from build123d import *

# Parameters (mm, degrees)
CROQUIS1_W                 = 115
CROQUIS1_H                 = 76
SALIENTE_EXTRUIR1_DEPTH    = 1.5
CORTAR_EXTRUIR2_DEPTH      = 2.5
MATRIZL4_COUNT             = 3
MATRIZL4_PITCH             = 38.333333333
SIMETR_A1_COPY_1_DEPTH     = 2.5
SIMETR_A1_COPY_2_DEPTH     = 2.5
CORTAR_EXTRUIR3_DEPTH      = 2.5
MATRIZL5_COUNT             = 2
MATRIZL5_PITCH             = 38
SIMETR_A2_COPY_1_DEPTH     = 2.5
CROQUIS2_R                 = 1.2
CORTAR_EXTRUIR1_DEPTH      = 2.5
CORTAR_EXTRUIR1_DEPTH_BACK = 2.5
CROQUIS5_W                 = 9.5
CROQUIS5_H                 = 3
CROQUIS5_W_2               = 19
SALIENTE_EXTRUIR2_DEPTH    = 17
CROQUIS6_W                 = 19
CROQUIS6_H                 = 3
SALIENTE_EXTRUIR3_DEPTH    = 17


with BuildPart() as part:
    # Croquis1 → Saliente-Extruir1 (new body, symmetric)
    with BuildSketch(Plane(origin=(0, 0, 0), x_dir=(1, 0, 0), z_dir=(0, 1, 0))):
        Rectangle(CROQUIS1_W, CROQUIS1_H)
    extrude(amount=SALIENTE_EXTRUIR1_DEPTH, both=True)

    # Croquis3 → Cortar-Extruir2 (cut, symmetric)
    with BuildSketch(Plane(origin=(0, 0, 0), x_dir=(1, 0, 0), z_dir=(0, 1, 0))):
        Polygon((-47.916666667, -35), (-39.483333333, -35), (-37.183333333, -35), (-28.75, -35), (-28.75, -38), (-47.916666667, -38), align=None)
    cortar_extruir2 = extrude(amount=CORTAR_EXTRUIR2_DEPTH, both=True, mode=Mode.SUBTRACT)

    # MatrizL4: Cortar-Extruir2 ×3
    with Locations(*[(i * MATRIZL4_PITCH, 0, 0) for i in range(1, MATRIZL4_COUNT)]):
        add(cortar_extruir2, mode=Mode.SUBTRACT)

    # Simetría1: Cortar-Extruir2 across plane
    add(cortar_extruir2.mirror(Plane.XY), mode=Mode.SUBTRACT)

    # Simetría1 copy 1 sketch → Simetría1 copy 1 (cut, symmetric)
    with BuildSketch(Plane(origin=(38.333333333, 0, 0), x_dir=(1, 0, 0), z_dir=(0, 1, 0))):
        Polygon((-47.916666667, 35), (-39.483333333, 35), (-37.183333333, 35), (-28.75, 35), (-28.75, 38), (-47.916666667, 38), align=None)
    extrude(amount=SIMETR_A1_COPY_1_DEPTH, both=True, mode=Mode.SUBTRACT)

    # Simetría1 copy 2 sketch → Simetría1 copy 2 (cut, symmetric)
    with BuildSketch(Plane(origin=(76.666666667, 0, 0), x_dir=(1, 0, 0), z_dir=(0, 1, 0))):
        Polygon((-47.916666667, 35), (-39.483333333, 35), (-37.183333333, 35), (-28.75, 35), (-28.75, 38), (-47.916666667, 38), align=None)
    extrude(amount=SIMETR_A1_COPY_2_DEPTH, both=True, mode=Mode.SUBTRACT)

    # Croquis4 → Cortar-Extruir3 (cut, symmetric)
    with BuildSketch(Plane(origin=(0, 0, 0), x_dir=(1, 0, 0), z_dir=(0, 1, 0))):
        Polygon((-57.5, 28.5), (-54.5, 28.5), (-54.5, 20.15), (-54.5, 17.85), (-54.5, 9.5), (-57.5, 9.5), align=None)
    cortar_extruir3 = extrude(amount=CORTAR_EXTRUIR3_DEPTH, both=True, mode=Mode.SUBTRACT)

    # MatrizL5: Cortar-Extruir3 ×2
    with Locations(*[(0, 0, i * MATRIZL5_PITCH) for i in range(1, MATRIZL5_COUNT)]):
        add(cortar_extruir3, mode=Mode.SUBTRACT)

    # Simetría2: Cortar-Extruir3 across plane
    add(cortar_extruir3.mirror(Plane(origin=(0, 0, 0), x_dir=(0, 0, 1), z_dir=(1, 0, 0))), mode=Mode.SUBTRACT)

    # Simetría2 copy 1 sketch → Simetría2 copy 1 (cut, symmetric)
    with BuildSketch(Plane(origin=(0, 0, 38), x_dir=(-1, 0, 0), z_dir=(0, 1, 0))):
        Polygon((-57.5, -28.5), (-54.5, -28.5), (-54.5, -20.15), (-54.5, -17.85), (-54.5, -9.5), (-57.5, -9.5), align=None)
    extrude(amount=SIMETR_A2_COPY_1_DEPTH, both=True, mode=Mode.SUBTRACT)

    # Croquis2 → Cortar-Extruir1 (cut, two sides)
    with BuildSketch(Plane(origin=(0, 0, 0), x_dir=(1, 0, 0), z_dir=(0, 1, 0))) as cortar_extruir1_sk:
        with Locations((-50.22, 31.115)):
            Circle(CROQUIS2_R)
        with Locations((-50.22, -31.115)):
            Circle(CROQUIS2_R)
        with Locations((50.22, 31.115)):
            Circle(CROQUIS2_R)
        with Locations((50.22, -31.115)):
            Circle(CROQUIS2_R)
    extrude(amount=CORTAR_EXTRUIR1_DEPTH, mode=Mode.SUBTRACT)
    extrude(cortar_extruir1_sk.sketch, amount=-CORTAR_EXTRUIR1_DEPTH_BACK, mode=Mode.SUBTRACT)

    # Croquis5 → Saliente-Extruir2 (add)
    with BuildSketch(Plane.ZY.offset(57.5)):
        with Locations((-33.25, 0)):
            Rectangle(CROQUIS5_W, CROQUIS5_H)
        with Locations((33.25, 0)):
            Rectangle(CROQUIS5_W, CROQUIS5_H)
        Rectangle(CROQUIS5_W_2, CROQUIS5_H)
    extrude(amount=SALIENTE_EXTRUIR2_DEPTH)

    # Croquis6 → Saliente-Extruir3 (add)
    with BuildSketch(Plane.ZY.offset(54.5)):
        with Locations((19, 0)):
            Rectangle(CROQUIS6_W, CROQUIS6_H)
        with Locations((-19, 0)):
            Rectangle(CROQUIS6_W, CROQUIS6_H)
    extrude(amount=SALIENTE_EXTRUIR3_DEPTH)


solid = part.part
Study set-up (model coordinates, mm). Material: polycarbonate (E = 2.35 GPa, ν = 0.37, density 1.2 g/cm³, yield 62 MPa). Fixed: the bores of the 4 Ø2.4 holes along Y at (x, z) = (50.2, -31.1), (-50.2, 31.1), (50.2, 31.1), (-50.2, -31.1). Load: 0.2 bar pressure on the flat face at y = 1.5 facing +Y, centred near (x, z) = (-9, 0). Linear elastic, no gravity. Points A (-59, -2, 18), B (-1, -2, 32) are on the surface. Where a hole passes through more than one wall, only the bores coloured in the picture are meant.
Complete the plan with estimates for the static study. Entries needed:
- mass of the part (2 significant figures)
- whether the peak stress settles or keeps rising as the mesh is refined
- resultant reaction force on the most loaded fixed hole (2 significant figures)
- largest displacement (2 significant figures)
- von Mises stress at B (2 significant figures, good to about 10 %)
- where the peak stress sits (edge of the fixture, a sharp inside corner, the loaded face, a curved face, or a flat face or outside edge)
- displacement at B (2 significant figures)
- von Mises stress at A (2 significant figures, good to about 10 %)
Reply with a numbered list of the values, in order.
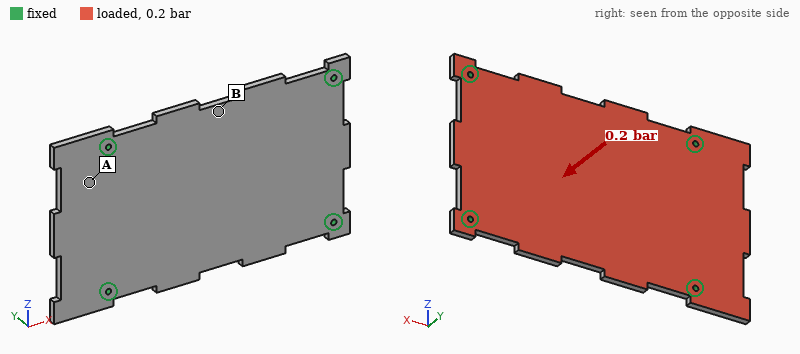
1. 34 g
2. keeps rising
3. 55 N
4. 1.6 mm
5. 8.3 MPa
6. edge of the fixture
7. 1.6 mm
8. 3.1 MPa
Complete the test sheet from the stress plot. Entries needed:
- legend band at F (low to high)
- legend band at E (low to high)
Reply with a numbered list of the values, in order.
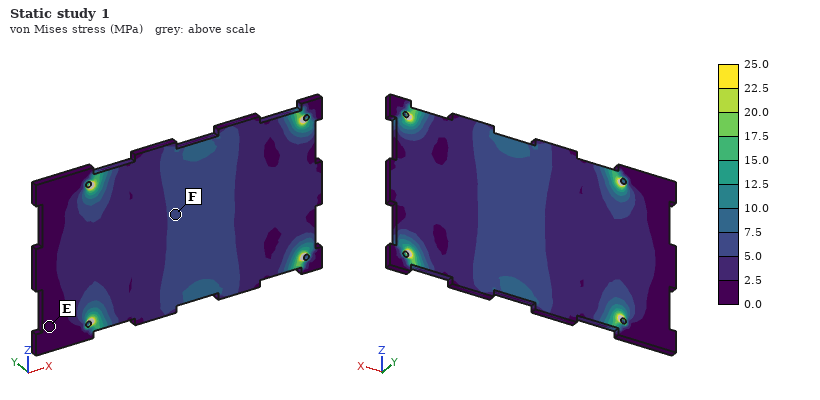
1. 5.0 to 7.5 MPa
2. 0.0 to 2.5 MPa
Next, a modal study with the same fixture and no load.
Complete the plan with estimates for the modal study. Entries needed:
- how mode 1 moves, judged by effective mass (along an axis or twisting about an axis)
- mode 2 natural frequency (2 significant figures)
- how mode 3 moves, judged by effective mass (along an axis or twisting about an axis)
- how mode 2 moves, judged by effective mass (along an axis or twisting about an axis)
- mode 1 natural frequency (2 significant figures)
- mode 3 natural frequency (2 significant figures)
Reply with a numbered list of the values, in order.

1. along Y
2. 540 Hz
3. along Y
4. twisting about X
5. 330 Hz
6. 740 Hz
